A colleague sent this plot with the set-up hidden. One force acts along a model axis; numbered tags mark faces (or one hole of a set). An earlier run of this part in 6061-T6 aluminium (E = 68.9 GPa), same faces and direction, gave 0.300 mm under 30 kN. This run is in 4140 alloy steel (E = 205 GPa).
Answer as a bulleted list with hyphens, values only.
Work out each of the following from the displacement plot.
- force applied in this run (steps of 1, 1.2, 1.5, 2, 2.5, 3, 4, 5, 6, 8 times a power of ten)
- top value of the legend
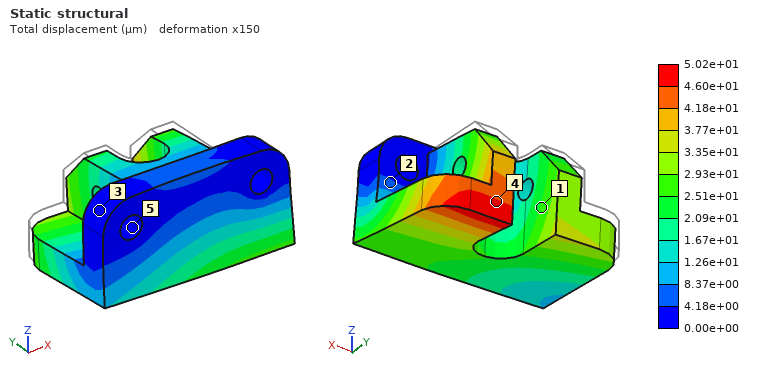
- 15 kN
- 5.02e+01 µm
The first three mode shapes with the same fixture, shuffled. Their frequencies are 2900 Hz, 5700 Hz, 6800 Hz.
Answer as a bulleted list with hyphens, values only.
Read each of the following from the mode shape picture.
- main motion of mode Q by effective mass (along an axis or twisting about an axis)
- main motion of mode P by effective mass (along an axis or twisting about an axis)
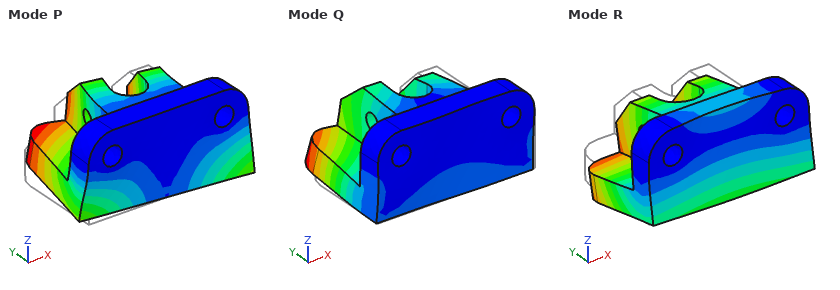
- along X
- along X
